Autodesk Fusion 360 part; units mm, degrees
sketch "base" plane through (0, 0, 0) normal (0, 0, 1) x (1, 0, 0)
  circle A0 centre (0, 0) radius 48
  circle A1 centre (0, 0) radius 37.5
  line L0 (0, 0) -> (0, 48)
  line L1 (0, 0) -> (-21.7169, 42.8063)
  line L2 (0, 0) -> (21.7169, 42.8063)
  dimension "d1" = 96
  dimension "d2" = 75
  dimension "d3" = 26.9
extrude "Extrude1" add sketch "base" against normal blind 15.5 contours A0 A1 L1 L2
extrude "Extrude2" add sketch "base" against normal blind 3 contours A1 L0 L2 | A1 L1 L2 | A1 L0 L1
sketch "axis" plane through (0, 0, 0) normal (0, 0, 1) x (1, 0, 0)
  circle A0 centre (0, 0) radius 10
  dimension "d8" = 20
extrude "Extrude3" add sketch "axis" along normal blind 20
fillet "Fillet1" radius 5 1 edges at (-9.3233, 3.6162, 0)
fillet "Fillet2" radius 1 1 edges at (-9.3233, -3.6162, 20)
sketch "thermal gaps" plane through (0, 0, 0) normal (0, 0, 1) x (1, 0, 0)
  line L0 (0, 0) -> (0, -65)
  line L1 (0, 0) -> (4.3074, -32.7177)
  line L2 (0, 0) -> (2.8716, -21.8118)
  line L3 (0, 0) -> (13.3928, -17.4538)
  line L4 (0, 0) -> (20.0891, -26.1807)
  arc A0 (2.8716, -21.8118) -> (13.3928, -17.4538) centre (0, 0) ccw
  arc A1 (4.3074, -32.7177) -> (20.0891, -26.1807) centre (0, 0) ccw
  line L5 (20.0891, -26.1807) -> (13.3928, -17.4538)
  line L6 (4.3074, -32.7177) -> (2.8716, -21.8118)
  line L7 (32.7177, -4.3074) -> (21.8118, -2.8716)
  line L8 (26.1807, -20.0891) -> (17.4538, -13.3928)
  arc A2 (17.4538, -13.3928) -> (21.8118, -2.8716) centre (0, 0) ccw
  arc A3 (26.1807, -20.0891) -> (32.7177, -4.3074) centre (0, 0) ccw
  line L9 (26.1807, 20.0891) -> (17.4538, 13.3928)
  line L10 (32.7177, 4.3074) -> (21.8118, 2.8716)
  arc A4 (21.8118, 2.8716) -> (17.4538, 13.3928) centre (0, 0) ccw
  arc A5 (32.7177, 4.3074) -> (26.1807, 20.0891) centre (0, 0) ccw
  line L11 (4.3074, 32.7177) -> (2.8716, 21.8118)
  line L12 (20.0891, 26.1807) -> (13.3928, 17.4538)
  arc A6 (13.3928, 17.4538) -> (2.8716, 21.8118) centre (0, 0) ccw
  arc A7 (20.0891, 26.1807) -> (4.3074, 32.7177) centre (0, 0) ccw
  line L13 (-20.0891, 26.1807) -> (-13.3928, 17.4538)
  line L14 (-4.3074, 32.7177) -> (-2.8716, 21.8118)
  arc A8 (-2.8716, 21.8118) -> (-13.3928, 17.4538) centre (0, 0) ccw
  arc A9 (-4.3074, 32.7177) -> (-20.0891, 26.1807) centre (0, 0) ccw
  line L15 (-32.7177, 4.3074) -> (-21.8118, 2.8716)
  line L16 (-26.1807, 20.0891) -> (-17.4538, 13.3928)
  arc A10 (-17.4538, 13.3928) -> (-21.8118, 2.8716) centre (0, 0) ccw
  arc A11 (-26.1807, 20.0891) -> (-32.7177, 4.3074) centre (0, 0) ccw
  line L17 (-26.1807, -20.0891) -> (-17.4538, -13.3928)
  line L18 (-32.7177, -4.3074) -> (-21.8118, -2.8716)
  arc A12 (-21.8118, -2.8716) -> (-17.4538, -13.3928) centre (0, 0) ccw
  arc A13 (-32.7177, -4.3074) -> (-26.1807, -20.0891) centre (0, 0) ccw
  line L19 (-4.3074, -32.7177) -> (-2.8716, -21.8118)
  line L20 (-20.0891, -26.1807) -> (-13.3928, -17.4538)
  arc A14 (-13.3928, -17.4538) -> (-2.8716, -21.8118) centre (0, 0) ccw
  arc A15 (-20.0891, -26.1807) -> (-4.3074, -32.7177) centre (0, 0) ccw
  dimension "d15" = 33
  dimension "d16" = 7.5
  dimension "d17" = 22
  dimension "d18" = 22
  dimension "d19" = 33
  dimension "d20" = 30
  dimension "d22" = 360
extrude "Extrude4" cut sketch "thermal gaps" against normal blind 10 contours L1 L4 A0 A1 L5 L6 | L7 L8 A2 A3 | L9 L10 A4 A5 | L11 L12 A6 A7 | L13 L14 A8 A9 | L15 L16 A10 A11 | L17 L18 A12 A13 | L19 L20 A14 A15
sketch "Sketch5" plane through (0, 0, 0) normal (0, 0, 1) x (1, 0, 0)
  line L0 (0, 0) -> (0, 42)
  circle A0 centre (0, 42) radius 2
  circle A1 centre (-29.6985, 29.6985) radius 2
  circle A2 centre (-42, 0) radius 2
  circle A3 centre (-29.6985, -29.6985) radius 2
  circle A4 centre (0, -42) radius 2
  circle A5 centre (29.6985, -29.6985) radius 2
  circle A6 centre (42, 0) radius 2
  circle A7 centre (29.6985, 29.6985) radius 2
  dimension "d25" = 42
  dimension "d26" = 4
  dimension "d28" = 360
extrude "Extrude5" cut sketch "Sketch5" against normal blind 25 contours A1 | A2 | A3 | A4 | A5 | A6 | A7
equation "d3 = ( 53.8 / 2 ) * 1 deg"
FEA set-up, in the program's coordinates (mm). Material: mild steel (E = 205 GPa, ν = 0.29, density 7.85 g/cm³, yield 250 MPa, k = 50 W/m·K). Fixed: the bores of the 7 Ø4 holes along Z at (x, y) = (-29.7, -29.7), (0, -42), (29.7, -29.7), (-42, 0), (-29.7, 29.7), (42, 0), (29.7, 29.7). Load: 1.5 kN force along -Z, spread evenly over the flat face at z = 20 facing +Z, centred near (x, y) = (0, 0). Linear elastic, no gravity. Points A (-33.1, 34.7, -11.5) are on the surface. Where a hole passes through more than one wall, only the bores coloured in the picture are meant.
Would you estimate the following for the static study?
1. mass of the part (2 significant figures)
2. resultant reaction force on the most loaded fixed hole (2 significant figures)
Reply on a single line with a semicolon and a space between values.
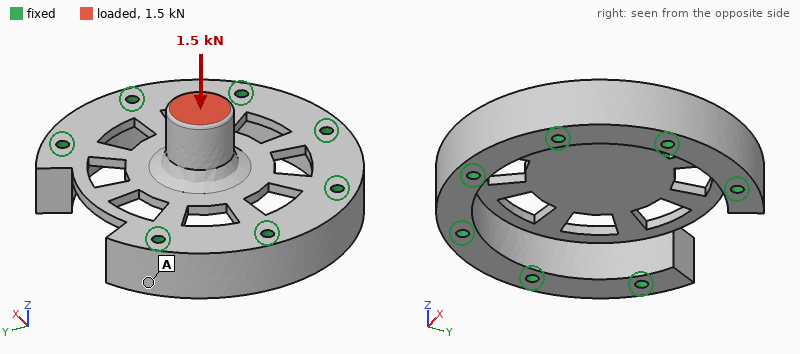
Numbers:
410 g; 340 N
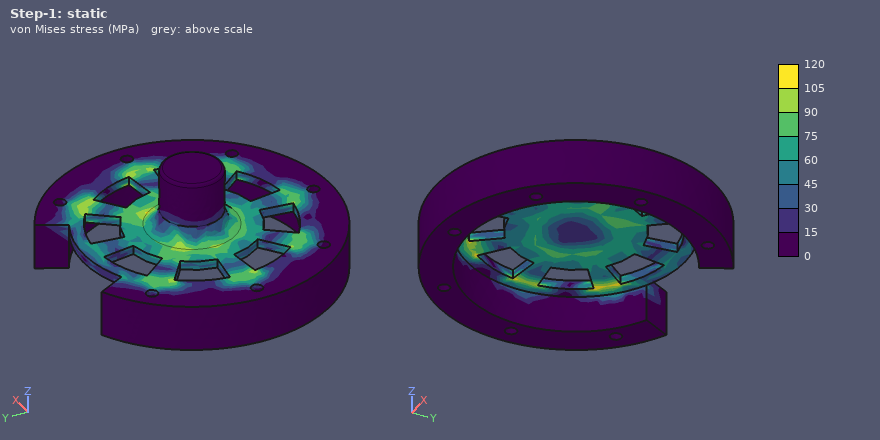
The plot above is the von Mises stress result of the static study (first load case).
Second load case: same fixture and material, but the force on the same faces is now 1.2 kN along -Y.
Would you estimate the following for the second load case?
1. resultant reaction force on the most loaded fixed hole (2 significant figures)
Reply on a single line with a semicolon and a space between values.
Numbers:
410 N
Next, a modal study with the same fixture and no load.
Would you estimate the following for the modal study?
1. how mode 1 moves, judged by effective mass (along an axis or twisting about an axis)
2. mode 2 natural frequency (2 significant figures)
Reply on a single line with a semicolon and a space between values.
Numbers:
along Z; 4300 Hz
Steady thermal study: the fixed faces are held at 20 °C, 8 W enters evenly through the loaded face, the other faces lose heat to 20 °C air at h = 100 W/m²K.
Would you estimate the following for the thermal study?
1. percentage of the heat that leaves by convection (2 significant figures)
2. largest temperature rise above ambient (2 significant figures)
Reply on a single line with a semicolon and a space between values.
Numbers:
65 %; 20 K
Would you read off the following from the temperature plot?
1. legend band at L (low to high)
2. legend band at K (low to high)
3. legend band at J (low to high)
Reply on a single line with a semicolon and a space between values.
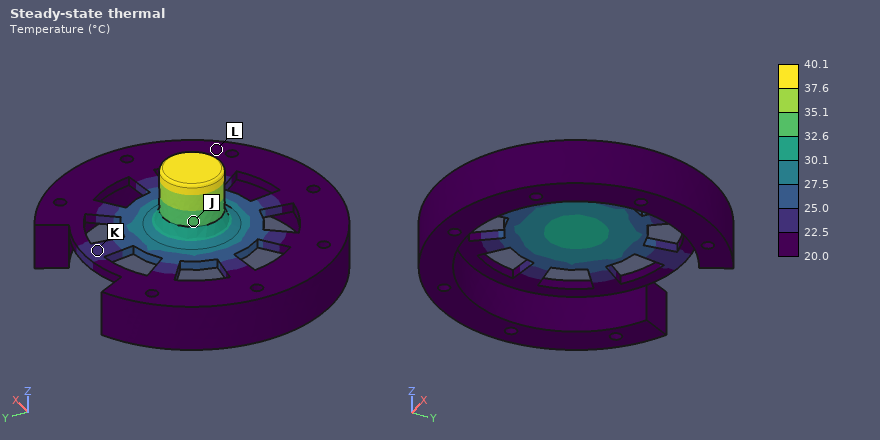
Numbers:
20.0 to 22.5 °C; 22.5 to 25.0 °C; 32.6 to 35.1 °C
